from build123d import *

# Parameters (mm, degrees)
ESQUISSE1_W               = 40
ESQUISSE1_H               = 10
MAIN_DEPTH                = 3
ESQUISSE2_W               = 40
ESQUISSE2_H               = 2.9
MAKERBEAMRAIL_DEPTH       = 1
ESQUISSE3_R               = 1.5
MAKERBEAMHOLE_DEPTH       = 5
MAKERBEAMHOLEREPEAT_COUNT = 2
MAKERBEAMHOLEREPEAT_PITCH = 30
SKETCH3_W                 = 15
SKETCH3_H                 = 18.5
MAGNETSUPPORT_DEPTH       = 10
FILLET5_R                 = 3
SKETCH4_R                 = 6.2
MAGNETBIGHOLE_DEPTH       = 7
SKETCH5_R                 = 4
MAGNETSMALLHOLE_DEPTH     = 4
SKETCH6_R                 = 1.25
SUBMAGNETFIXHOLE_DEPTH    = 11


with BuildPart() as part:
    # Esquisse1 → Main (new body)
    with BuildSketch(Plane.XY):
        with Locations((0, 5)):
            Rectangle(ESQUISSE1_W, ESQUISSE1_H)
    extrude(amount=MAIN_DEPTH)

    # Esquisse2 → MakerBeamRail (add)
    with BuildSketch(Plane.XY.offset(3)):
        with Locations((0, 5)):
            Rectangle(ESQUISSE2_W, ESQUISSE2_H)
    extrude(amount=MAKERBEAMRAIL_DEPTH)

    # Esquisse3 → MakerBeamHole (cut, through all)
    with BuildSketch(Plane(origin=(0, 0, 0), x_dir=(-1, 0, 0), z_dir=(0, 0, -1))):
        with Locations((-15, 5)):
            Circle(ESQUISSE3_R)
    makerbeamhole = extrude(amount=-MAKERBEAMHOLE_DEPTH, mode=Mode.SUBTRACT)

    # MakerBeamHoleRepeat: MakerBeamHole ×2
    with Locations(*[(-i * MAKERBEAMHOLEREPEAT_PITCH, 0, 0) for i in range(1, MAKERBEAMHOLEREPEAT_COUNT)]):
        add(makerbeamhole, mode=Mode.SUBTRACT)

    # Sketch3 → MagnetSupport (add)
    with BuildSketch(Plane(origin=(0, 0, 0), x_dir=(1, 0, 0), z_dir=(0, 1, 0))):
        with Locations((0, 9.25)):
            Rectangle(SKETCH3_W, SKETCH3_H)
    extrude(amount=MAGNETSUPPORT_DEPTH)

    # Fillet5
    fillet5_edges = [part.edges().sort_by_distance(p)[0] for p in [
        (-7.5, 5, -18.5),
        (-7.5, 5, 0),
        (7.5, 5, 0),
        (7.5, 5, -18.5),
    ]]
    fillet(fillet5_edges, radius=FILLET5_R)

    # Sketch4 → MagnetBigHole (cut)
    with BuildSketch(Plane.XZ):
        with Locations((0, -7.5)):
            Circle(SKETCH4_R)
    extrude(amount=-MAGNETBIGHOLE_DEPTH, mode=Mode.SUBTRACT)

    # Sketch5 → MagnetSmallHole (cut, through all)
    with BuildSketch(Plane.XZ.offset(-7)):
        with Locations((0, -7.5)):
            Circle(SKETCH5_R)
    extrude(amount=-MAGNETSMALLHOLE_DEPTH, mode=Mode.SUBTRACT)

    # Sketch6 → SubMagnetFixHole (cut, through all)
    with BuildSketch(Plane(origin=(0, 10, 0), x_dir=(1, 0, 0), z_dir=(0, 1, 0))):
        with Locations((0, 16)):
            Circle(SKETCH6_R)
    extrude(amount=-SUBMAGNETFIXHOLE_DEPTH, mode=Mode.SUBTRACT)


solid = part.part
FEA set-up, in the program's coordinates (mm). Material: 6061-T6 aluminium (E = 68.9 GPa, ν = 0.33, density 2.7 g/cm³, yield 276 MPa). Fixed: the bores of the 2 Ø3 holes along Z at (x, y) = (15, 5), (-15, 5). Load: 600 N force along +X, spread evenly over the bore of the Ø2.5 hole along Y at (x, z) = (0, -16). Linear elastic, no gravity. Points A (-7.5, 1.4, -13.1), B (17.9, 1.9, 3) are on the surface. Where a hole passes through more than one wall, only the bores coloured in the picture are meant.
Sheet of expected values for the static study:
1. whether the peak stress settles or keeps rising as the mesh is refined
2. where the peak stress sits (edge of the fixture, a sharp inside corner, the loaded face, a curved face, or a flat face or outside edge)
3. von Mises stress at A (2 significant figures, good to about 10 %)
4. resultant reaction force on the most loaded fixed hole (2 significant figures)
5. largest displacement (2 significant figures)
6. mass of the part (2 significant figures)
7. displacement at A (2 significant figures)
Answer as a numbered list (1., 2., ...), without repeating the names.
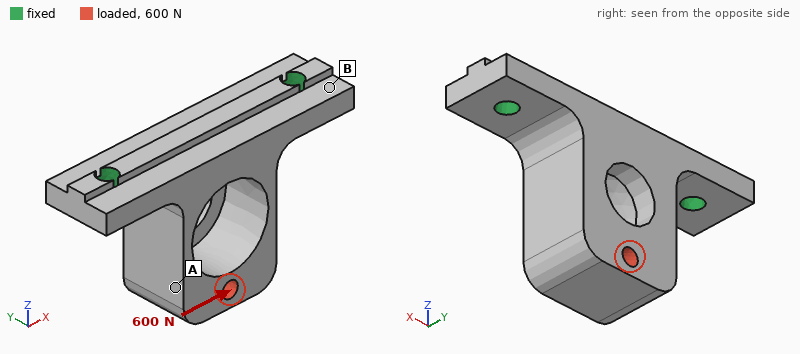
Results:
1. keeps rising
2. edge of the fixture
3. 18 MPa
4. 550 N
5. 61 µm
6. 8.1 g
7. 51 µm
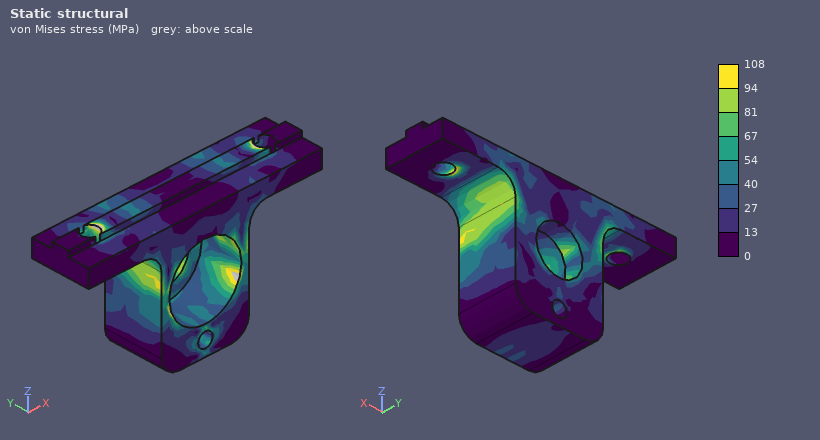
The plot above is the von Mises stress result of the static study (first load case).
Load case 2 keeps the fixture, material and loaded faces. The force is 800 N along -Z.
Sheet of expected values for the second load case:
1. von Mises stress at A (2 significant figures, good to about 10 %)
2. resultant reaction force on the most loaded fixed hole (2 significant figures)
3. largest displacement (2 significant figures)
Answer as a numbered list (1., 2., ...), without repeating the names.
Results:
1. 15 MPa
2. 460 N
3. 21 µm
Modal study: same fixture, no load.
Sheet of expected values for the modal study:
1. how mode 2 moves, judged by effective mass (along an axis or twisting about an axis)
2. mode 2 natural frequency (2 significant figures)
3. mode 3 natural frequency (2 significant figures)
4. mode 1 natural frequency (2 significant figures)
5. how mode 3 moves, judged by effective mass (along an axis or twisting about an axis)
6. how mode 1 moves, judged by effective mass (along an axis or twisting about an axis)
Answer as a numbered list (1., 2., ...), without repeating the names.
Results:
1. along X
2. 11 kHz
3. 16 kHz
4. 4800 Hz
5. along Z
6. along Y
